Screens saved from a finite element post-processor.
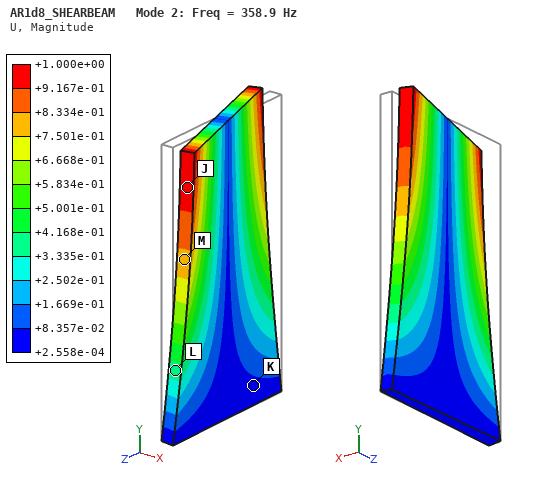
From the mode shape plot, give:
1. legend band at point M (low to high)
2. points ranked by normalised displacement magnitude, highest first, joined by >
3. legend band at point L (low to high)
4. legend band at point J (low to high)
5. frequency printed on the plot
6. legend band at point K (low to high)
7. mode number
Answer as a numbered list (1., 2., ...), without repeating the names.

1. +7.501e-01 to +8.334e-01
2. J > M > L > K
3. +3.335e-01 to +4.168e-01
4. +9.167e-01 to +1.000e+00
5. 358.9 Hz
6. +2.558e-04 to +8.357e-02
7. 2
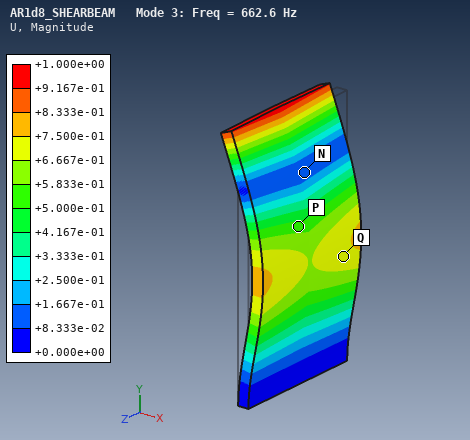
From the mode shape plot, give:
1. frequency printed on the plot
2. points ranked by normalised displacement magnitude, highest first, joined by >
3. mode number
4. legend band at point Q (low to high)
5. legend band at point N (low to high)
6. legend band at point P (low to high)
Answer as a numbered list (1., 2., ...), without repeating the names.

1. 662.6 Hz
2. Q > P > N
3. 3
4. +6.667e-01 to +7.500e-01
5. +8.333e-02 to +1.667e-01
6. +5.000e-01 to +5.833e-01
